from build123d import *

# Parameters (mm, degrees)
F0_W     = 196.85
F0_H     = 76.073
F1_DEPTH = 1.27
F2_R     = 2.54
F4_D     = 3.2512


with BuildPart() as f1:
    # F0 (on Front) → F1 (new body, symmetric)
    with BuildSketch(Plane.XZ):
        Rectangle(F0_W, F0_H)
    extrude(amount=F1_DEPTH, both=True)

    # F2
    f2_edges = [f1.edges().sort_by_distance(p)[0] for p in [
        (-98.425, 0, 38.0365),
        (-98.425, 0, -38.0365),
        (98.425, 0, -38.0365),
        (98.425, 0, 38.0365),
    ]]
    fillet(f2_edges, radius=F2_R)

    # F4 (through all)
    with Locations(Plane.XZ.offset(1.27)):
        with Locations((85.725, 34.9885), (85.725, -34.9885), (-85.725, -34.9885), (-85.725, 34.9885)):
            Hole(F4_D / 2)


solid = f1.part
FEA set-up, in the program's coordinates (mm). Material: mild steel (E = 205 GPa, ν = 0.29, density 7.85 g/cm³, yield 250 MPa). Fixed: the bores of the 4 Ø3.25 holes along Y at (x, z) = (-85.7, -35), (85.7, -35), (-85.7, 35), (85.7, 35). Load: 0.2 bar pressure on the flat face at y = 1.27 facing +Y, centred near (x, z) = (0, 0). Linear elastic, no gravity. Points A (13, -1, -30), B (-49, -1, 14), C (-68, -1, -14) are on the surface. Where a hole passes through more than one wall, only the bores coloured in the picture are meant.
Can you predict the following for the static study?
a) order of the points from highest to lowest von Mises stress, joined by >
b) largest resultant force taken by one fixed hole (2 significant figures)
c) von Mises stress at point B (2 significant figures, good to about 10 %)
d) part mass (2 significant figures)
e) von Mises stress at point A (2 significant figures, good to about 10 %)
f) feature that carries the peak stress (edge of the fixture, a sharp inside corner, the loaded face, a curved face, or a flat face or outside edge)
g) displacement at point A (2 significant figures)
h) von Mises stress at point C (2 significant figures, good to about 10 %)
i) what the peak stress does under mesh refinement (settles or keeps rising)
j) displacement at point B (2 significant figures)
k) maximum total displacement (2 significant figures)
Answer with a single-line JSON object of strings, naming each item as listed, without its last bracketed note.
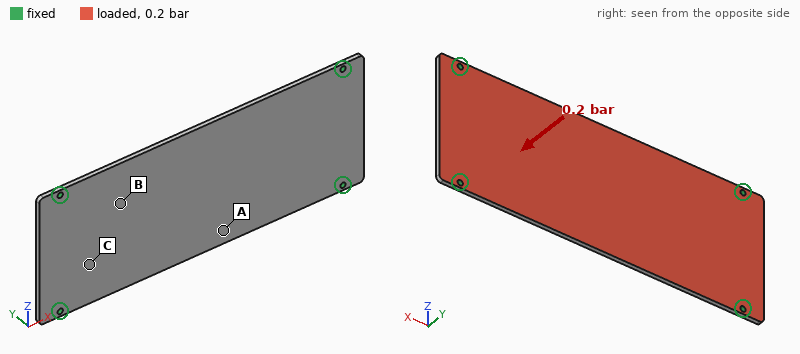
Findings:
{"order of the points from highest to lowest von Mises stress, joined by >": "A > C > B", "largest resultant force taken by one fixed hole": "75 N", "von Mises stress at point B": "7.3 MPa", "part mass": "300 g", "von Mises stress at point A": "26 MPa", "feature that carries the peak stress": "edge of the fixture", "displacement at point A": "0.21 mm", "von Mises stress at point C": "16 MPa", "what the peak stress does under mesh refinement": "keeps rising", "displacement at point B": "0.12 mm", "maximum total displacement": "0.23 mm"}
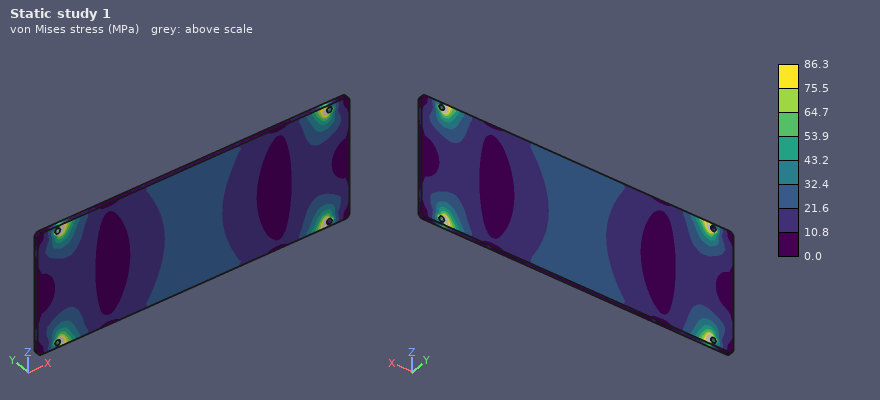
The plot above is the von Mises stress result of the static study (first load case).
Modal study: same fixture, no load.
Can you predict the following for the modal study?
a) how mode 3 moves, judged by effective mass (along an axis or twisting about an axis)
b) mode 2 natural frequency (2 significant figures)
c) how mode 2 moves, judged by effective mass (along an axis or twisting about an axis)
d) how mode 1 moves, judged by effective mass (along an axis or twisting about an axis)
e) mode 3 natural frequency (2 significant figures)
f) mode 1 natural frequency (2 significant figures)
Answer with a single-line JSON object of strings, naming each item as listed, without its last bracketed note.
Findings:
{"how mode 3 moves, judged by effective mass": "twisting about Z", "mode 2 natural frequency": "800 Hz", "how mode 2 moves, judged by effective mass": "twisting about X", "how mode 1 moves, judged by effective mass": "along Y", "mode 3 natural frequency": "1100 Hz", "mode 1 natural frequency": "380 Hz"}
